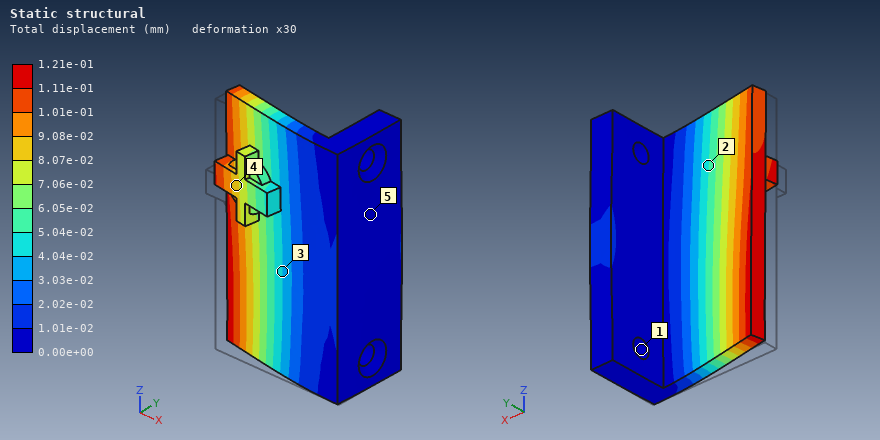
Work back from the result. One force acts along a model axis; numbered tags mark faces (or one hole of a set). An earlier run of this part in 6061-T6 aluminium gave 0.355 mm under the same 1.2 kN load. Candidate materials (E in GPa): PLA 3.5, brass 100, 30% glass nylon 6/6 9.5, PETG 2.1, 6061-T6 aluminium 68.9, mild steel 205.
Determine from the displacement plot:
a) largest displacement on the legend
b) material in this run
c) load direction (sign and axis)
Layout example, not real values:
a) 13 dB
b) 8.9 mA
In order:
a) 1.21e-01 mm
b) mild steel
c) +Y
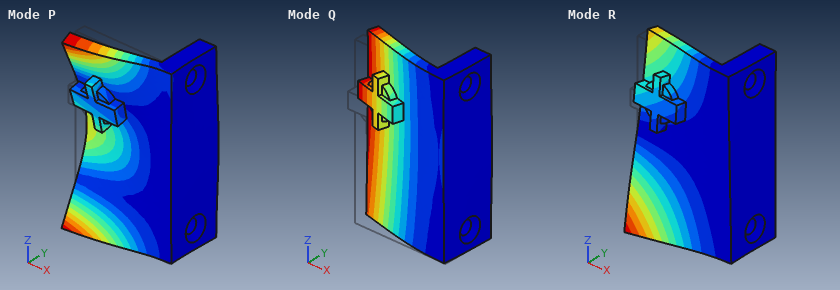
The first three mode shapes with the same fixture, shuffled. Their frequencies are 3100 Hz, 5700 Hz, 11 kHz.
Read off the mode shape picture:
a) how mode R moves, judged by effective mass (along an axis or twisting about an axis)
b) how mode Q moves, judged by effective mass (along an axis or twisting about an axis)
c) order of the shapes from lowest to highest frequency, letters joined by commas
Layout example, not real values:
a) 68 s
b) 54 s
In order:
a) twisting about X
b) along Y
c) Q, R, P
